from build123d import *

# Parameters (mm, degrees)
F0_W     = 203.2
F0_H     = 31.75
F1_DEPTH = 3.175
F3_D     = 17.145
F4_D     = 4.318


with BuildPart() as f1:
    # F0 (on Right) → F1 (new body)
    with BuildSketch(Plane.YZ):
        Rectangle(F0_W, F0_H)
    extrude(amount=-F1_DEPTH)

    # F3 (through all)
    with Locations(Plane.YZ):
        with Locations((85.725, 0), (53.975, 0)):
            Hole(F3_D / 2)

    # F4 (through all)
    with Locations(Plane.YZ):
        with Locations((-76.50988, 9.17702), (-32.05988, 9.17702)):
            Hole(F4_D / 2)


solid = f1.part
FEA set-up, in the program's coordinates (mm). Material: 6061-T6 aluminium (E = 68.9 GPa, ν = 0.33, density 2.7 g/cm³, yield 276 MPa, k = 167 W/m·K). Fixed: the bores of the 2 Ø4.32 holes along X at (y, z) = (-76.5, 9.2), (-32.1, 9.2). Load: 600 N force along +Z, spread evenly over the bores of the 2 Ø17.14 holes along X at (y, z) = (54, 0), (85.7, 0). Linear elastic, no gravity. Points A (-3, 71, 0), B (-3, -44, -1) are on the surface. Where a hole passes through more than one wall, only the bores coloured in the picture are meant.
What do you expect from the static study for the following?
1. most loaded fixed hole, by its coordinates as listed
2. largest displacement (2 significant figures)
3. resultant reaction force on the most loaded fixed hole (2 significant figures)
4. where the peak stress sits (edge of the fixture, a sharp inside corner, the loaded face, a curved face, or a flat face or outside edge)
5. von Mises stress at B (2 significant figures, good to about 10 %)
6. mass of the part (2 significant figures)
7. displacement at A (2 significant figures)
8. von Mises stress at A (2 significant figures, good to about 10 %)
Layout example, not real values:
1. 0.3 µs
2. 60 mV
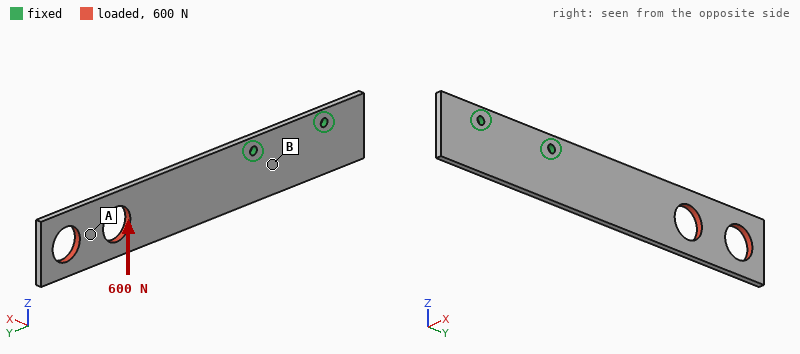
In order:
1. (-32.1, 9.2)
2. 0.80 mm
3. 2.2 kN
4. edge of the fixture
5. 35 MPa
6. 51 g
7. 0.57 mm
8. 18 MPa
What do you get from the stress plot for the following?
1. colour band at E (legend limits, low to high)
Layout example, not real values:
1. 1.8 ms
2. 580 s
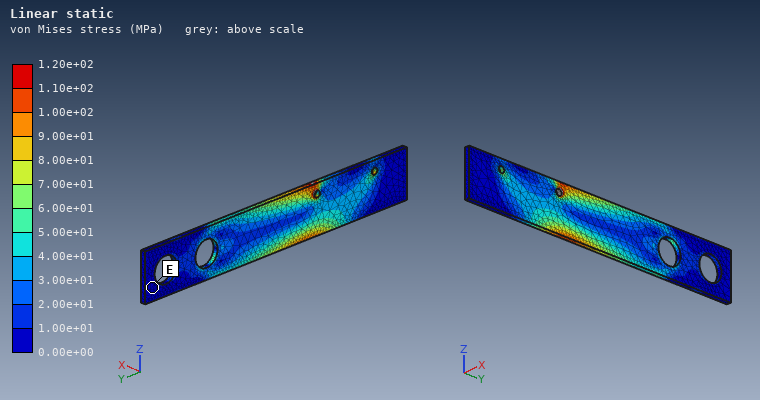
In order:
1. 0.00e+00 to 1.00e+01 MPa
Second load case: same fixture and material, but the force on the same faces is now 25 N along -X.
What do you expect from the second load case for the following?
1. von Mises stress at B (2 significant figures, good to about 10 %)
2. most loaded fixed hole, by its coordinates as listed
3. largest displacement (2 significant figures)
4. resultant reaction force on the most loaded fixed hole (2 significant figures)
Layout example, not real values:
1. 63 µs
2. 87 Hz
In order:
1. 7.6 MPa
2. (-32.1, 9.2)
3. 2.4 mm
4. 43 N
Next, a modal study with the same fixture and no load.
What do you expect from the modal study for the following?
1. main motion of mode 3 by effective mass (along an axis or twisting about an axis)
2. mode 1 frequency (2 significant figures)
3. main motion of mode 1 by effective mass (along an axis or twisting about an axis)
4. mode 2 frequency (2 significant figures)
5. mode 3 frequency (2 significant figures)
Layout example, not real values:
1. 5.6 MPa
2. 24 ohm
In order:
1. twisting about Y
2. 160 Hz
3. along X
4. 840 Hz
5. 1100 Hz
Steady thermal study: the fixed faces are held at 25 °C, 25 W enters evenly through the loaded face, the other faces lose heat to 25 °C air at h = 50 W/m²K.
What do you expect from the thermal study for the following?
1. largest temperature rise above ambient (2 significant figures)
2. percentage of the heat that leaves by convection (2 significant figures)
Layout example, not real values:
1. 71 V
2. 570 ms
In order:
1. 79 K
2. 70 %
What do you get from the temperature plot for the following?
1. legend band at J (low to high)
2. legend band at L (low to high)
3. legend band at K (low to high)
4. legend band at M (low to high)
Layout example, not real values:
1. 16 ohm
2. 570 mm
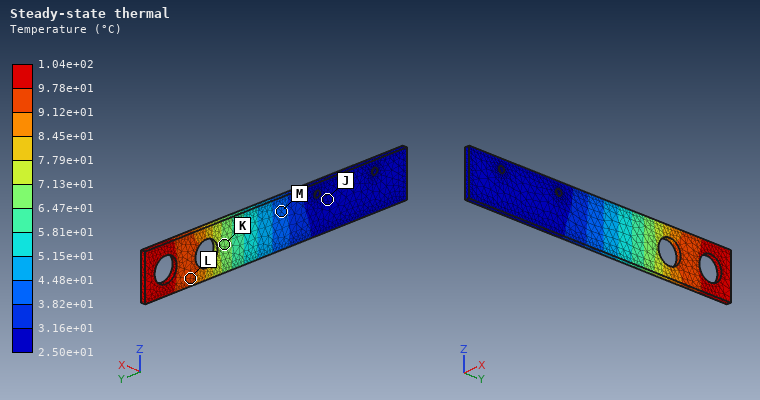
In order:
1. 2.50e+01 to 3.16e+01 °C
2. 9.12e+01 to 9.78e+01 °C
3. 6.47e+01 to 7.13e+01 °C
4. 3.82e+01 to 4.48e+01 °C
